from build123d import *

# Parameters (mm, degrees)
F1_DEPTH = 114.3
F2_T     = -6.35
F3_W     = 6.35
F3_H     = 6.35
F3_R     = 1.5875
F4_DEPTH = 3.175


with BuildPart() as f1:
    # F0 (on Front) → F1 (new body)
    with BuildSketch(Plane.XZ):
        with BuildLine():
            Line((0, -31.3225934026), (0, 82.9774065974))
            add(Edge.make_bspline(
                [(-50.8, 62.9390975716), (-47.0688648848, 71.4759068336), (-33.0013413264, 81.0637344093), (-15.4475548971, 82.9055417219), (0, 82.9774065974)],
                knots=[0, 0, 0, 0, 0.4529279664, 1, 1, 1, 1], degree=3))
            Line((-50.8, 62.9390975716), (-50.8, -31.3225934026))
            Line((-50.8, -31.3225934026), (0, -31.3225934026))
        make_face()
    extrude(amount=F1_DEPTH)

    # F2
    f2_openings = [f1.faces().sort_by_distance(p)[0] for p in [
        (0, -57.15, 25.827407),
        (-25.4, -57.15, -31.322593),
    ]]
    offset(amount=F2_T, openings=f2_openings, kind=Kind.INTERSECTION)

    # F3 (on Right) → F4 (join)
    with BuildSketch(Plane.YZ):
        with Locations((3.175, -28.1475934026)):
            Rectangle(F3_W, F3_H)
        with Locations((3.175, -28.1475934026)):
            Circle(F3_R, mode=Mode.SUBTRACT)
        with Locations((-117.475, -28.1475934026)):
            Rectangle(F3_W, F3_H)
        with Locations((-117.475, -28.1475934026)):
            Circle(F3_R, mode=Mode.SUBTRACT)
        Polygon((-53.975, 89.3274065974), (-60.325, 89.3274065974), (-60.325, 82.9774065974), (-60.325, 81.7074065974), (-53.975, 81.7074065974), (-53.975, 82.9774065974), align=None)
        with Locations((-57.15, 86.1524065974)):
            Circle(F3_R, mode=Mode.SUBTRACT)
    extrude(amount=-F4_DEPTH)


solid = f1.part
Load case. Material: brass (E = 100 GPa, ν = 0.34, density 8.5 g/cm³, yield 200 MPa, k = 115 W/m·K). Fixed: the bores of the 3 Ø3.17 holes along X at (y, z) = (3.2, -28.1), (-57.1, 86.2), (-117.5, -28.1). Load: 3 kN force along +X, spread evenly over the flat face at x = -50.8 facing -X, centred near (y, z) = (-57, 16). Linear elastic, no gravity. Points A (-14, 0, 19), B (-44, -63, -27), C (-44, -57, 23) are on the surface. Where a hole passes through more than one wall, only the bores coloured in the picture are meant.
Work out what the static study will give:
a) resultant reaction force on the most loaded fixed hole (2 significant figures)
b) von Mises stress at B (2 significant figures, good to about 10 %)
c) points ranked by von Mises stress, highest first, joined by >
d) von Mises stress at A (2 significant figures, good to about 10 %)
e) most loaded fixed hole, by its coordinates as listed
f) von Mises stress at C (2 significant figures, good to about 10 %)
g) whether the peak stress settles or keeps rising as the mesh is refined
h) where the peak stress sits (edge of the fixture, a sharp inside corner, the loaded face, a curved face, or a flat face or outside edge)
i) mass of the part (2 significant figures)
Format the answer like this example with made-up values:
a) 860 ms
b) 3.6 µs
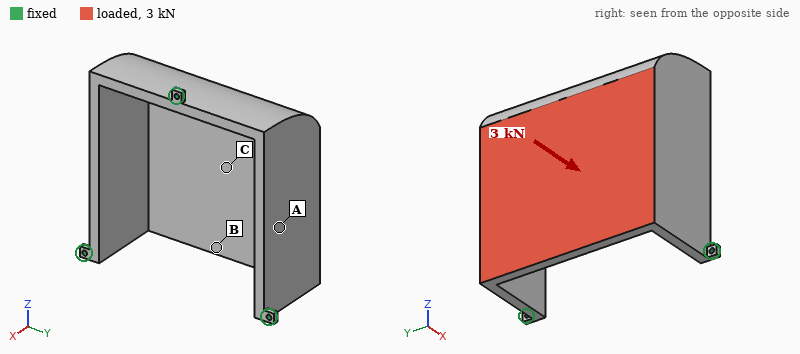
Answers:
a) 1.3 kN
b) 26 MPa
c) B > C > A
d) 6.6 MPa
e) (-57.1, 86.2)
f) 15 MPa
g) keeps rising
h) edge of the fixture
i) 1.4 kg
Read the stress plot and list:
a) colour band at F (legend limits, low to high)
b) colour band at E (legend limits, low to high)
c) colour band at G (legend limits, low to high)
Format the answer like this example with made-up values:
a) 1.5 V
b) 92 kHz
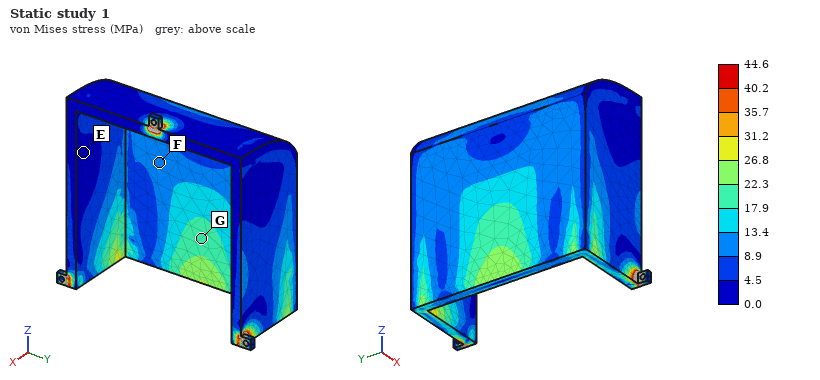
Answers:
a) 8.9 to 13.4 MPa
b) 0.0 to 4.5 MPa
c) 17.9 to 22.3 MPa
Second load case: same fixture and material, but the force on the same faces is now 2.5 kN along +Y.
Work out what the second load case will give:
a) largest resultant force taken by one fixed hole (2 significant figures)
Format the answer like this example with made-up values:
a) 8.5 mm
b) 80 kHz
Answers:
a) 1.4 kN
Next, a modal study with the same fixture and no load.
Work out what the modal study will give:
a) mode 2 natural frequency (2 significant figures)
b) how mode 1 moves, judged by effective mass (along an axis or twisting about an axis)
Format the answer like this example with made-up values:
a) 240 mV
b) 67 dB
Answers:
a) 1400 Hz
b) along Y
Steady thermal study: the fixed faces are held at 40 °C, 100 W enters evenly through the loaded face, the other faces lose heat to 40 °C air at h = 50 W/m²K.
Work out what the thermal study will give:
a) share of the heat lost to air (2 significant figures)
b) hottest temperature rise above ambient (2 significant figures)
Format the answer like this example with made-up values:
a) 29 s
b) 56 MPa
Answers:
a) 73 %
b) 48 K
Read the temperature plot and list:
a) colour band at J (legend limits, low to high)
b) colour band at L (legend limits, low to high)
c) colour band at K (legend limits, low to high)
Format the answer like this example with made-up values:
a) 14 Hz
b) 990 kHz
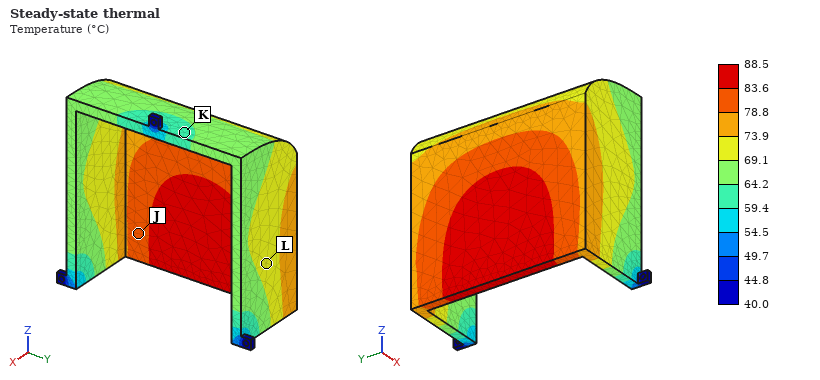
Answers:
a) 78.8 to 83.6 °C
b) 69.1 to 73.9 °C
c) 59.4 to 64.2 °C
